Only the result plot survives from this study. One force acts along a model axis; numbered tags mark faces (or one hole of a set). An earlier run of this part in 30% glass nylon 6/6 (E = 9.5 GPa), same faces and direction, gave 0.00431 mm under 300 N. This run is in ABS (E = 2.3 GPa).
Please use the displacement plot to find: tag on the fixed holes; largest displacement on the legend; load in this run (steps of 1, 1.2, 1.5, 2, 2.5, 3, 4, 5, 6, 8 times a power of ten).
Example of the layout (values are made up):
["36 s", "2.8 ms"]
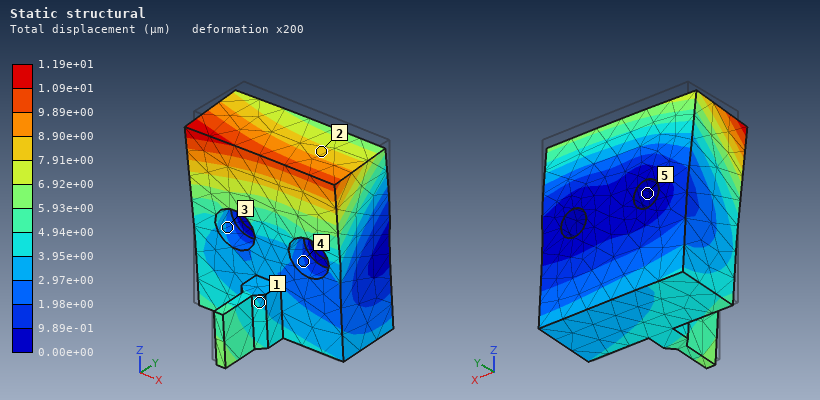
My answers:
["5", "1.19e+01 µm", "200 N"]
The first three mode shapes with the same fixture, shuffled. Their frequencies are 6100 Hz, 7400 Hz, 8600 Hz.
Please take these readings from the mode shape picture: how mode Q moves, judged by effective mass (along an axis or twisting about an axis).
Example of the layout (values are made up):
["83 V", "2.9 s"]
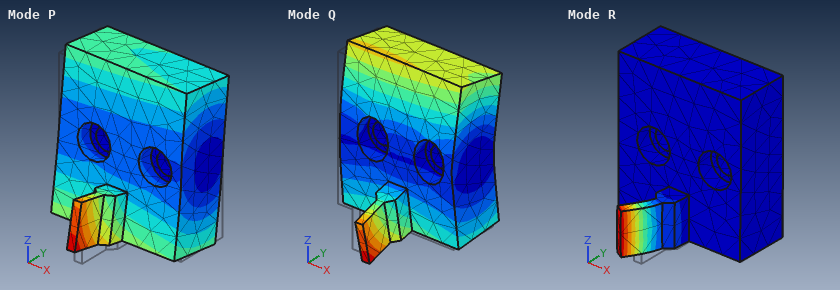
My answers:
["along Y"]
